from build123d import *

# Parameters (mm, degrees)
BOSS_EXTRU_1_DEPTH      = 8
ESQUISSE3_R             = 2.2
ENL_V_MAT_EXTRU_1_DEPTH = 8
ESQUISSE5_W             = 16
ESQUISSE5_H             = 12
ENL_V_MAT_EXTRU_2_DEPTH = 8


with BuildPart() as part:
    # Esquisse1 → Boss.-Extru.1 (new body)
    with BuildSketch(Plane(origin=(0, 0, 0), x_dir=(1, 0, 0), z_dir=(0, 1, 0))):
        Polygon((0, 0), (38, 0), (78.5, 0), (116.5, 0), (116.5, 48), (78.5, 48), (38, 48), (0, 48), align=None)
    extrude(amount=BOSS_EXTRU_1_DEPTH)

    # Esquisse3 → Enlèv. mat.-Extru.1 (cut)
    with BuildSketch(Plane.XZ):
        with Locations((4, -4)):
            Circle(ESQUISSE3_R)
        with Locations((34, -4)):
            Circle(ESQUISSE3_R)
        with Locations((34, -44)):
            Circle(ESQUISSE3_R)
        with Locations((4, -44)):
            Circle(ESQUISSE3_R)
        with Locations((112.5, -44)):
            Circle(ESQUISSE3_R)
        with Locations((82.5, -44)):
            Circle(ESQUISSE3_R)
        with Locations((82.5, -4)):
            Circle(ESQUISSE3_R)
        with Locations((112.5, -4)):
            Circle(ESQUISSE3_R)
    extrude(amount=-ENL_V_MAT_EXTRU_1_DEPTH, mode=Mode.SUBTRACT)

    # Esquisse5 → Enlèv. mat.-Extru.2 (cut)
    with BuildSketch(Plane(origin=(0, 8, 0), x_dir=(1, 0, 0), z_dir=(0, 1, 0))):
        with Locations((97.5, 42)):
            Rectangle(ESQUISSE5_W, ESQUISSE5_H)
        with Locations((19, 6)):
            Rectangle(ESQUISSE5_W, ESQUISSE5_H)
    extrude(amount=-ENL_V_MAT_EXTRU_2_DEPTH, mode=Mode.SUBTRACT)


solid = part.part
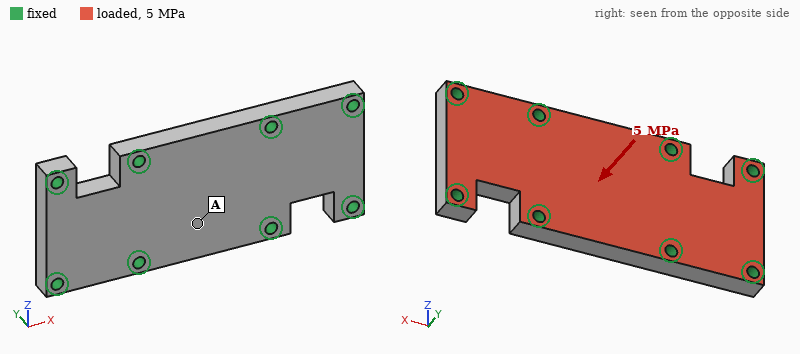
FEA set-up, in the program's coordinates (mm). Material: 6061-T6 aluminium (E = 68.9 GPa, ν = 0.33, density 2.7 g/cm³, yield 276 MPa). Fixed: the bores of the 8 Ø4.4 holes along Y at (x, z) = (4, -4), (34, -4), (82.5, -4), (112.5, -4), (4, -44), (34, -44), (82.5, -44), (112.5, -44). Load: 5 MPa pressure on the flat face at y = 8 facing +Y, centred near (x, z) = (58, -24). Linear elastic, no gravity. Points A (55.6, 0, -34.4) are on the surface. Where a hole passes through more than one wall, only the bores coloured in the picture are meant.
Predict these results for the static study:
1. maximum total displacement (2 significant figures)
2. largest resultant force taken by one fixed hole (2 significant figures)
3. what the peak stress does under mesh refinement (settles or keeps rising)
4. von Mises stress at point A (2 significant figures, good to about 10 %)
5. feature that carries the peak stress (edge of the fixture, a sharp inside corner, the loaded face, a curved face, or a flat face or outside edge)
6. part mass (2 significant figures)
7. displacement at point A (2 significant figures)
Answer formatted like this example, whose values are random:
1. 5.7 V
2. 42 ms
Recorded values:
1. 53 µm
2. 4.8 kN
3. keeps rising
4. 44 MPa
5. edge of the fixture
6. 110 g
7. 48 µm
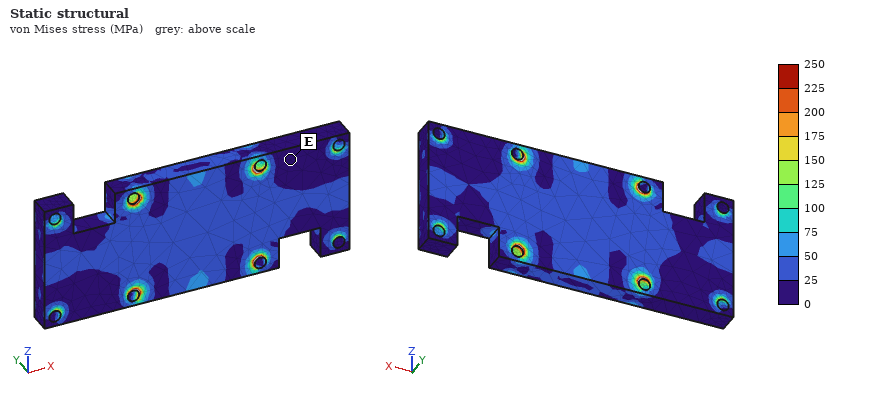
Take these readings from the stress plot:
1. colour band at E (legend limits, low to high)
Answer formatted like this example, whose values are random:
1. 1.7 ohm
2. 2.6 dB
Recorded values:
1. 0 to 25 MPa
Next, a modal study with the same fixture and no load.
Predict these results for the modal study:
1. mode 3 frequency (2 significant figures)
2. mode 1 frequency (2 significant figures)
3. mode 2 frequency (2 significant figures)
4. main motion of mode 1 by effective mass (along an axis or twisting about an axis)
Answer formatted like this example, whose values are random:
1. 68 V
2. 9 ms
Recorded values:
1. 18 kHz
2. 12 kHz
3. 18 kHz
4. along Y
